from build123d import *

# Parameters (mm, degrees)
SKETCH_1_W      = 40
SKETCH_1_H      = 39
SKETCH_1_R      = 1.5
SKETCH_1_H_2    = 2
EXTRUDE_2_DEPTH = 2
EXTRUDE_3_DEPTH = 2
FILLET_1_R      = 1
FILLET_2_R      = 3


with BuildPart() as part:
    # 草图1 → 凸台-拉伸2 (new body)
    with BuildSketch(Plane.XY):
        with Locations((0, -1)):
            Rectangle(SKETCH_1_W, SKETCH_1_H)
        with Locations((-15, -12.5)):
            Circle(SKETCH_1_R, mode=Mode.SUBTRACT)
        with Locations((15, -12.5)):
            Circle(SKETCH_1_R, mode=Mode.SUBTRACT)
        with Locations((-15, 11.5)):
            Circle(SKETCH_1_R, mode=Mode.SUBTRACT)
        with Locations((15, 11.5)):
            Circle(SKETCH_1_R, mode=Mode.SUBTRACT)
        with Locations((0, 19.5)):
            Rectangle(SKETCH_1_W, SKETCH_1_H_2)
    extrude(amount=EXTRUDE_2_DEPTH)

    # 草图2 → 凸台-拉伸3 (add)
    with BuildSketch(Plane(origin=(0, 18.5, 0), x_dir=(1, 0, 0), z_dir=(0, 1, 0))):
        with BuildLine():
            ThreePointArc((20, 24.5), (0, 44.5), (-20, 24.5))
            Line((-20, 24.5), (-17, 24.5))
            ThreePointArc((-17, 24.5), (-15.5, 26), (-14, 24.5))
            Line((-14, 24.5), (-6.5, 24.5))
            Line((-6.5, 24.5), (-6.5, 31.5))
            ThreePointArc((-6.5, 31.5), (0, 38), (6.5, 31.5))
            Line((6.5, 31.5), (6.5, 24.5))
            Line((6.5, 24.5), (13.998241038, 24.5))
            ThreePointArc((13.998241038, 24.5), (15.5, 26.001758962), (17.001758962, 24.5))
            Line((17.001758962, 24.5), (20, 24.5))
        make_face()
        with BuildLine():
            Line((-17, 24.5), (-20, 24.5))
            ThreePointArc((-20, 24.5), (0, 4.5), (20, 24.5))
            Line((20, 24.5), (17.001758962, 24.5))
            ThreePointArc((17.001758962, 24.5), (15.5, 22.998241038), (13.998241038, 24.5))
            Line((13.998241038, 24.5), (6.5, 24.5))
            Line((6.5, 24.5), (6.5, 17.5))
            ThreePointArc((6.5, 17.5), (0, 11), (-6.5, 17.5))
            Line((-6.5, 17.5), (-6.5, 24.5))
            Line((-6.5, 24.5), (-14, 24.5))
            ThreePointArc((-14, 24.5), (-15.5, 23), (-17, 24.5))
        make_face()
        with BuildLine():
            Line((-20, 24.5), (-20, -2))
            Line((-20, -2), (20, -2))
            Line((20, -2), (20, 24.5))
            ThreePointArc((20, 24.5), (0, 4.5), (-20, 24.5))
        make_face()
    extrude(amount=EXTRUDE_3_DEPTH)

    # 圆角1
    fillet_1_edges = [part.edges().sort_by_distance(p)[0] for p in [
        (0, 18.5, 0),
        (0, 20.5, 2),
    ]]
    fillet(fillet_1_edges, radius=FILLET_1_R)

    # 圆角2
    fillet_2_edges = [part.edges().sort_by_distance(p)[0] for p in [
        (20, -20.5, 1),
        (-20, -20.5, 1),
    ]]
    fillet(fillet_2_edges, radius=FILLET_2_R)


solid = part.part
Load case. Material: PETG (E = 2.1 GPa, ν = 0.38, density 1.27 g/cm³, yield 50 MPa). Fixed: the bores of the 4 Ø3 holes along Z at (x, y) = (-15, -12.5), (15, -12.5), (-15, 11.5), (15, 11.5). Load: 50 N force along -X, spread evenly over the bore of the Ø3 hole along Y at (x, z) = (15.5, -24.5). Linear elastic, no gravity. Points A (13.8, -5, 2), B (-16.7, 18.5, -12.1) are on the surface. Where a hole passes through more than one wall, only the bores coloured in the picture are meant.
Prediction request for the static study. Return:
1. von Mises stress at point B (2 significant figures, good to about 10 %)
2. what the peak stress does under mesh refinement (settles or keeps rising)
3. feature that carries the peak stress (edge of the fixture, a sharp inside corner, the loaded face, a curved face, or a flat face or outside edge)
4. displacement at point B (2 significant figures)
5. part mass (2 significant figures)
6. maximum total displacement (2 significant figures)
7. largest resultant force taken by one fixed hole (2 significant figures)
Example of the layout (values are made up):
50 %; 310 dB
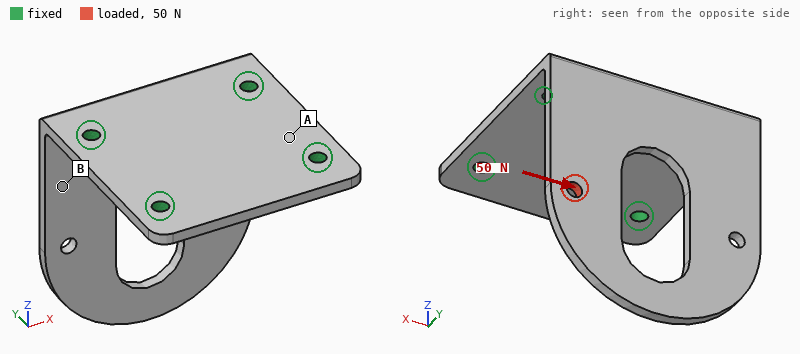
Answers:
3.9 MPa; keeps rising; edge of the fixture; 0.43 mm; 7.3 g; 0.81 mm; 52 N
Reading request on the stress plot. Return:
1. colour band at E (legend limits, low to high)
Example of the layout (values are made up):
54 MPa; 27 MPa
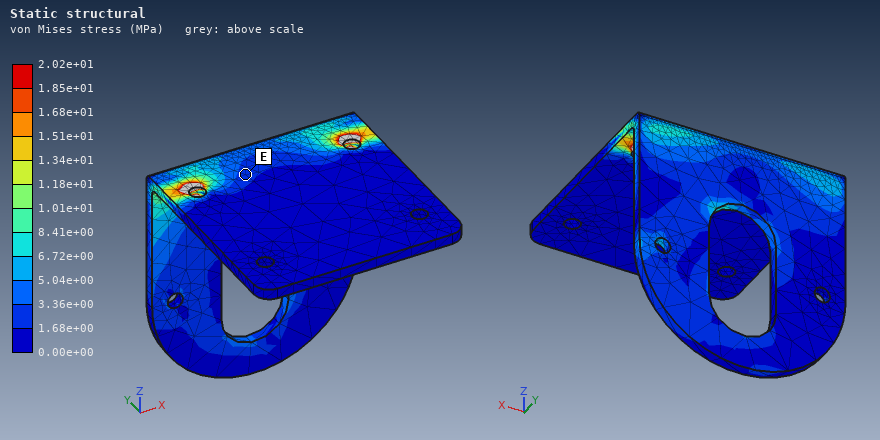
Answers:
1.68e+00 to 3.36e+00 MPa
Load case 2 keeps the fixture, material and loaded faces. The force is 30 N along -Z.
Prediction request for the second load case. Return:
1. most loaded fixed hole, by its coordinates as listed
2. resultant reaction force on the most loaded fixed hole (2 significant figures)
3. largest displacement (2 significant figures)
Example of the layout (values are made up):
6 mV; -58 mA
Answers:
(15, 11.5); 32 N; 0.87 mm
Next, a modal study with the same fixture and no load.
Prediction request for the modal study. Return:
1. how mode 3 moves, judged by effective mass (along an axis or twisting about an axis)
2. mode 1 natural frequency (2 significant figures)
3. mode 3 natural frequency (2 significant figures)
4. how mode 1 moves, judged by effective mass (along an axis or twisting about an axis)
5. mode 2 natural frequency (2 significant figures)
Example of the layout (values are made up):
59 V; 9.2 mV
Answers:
along X; 210 Hz; 1000 Hz; along Y; 550 Hz
